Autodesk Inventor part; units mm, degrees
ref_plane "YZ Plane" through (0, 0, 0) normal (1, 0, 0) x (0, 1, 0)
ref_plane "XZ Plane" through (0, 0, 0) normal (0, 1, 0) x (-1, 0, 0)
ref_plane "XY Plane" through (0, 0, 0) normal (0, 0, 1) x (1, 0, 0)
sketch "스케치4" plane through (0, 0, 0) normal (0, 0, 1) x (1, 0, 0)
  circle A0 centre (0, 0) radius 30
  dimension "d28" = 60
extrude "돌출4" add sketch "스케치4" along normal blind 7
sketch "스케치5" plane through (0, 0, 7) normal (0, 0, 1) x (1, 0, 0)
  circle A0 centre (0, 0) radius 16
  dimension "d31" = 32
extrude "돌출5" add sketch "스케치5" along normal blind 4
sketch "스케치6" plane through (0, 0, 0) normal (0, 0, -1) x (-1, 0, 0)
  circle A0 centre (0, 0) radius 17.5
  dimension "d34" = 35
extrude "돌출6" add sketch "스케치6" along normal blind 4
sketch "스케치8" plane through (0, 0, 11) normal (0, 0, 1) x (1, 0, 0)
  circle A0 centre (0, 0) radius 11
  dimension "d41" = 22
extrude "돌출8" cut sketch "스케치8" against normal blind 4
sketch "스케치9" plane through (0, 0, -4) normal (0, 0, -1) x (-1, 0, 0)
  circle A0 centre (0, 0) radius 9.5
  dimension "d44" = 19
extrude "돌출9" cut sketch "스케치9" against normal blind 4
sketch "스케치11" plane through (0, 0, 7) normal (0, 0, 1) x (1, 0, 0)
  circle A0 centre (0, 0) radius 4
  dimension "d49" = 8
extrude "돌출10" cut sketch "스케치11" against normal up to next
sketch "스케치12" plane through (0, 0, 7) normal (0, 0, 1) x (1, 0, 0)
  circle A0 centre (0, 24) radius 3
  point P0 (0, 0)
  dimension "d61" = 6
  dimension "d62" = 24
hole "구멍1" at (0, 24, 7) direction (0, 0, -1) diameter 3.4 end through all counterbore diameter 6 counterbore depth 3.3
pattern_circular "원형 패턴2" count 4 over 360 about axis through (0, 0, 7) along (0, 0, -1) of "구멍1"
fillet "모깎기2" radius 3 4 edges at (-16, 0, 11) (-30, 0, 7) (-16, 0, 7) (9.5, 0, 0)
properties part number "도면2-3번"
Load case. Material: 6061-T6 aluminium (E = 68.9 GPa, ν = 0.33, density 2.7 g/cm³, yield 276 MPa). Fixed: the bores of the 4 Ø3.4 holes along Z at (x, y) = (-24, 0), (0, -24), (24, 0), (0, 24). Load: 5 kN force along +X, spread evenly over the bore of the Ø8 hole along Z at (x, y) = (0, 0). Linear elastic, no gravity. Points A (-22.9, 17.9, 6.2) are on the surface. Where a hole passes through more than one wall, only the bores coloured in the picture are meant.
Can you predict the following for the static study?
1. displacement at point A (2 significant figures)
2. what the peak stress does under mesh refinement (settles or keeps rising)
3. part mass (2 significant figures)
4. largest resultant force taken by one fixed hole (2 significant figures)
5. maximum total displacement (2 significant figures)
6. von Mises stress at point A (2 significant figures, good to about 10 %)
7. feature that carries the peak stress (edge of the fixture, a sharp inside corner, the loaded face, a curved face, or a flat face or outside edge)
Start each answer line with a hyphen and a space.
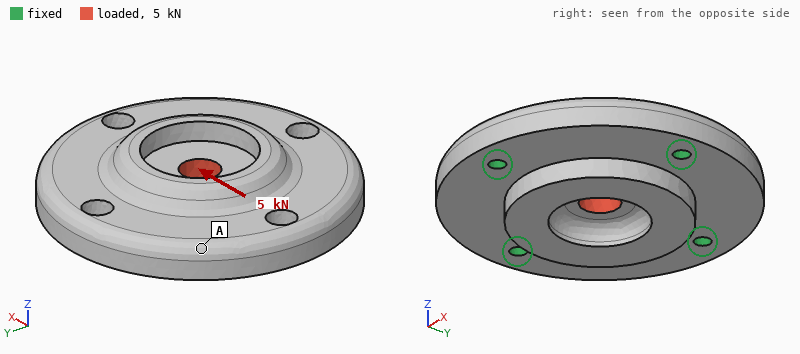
- 3.4 µm
- keeps rising
- 62 g
- 1.5 kN
- 7.3 µm
- 6.2 MPa
- edge of the fixture
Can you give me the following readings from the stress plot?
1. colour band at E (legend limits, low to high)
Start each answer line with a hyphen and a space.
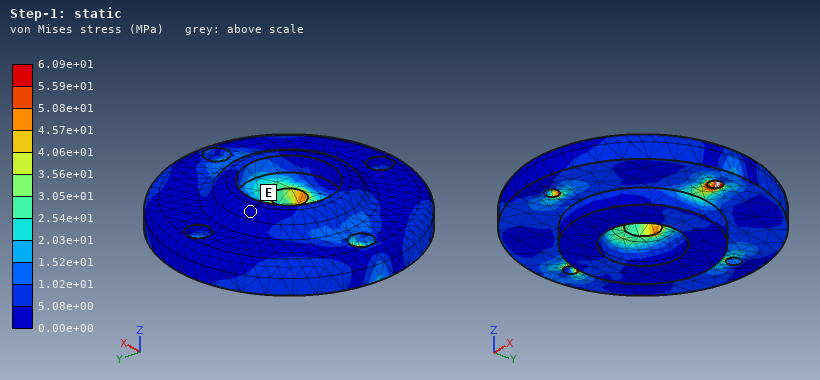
- 0.00e+00 to 5.08e+00 MPa
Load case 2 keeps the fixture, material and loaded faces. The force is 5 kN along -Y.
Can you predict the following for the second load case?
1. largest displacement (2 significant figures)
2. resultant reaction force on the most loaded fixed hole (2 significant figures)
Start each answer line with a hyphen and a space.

- 7.2 µm
- 1.5 kN
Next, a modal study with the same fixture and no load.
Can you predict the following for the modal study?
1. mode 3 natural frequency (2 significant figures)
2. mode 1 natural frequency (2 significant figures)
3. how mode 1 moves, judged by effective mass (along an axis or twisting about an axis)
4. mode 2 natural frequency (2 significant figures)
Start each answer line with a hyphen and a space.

- 18 kHz
- 16 kHz
- along Z
- 17 kHz
